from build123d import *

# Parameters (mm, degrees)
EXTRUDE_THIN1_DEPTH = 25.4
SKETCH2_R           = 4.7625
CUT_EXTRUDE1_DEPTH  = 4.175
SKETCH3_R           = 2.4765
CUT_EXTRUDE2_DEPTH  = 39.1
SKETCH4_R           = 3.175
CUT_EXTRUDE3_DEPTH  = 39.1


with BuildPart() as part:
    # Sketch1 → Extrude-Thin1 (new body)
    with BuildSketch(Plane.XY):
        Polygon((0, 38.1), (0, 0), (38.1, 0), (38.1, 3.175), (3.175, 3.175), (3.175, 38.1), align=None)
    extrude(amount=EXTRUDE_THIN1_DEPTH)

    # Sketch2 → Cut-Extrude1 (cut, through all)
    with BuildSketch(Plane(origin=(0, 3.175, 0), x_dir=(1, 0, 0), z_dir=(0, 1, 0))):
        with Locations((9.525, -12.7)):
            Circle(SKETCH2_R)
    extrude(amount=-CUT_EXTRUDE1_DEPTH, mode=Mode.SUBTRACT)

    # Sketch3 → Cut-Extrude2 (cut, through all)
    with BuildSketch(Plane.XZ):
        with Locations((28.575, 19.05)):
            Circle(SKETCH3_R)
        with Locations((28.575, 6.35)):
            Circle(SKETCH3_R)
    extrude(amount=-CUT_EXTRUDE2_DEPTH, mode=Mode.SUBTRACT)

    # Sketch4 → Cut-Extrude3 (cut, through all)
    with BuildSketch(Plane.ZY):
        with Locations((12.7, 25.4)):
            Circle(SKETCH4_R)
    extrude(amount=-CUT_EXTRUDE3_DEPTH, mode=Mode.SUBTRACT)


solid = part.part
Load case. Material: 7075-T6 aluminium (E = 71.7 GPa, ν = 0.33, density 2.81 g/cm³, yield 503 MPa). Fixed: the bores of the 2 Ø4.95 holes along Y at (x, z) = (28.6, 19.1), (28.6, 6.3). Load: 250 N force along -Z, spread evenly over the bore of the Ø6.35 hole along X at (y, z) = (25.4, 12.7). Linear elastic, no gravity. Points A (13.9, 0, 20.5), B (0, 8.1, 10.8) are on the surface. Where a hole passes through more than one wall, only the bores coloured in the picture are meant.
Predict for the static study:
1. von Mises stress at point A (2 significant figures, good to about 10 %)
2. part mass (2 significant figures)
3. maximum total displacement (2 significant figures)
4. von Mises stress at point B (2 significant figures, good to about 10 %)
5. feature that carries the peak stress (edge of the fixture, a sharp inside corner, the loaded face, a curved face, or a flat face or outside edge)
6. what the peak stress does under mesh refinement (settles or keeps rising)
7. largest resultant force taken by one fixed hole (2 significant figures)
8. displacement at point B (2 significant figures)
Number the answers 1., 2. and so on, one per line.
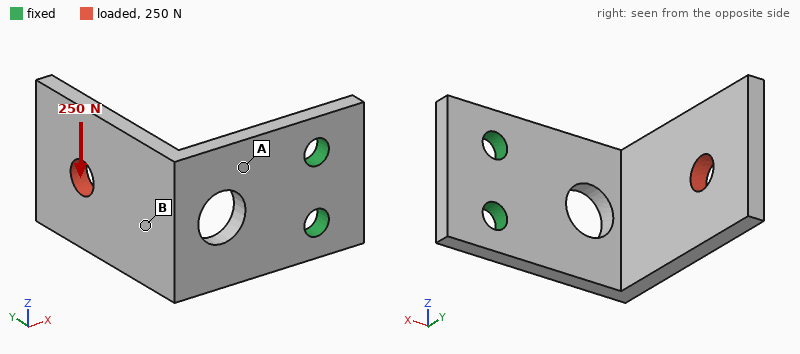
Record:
1. 110 MPa
2. 15 g
3. 0.69 mm
4. 24 MPa
5. edge of the fixture
6. keeps rising
7. 540 N
8. 0.13 mm
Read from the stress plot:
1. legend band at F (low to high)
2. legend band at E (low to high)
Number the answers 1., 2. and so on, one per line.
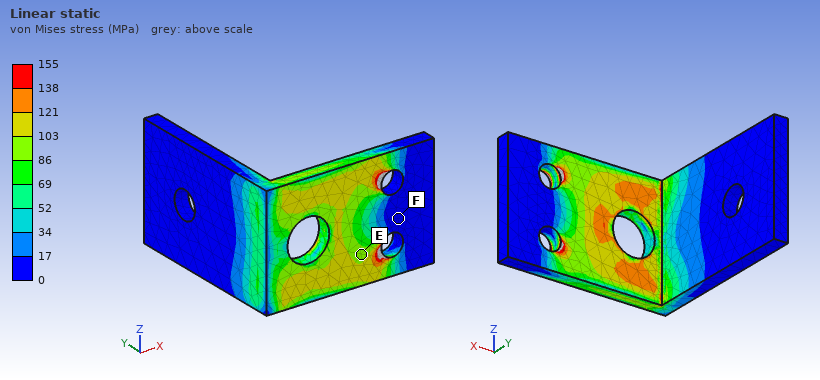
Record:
1. 0 to 17 MPa
2. 86 to 103 MPa
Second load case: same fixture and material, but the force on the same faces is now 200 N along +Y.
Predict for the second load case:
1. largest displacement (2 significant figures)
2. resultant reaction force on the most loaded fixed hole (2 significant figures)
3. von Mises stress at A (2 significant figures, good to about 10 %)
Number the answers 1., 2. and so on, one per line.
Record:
1. 0.61 mm
2. 100 N
3. 75 MPa
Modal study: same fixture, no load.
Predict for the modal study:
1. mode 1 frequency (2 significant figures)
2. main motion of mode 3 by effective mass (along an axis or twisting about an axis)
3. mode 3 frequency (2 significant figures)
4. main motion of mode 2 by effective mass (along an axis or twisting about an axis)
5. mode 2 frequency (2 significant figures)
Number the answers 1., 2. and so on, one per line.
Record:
1. 850 Hz
2. along Y
3. 2600 Hz
4. along Z
5. 1400 Hz
